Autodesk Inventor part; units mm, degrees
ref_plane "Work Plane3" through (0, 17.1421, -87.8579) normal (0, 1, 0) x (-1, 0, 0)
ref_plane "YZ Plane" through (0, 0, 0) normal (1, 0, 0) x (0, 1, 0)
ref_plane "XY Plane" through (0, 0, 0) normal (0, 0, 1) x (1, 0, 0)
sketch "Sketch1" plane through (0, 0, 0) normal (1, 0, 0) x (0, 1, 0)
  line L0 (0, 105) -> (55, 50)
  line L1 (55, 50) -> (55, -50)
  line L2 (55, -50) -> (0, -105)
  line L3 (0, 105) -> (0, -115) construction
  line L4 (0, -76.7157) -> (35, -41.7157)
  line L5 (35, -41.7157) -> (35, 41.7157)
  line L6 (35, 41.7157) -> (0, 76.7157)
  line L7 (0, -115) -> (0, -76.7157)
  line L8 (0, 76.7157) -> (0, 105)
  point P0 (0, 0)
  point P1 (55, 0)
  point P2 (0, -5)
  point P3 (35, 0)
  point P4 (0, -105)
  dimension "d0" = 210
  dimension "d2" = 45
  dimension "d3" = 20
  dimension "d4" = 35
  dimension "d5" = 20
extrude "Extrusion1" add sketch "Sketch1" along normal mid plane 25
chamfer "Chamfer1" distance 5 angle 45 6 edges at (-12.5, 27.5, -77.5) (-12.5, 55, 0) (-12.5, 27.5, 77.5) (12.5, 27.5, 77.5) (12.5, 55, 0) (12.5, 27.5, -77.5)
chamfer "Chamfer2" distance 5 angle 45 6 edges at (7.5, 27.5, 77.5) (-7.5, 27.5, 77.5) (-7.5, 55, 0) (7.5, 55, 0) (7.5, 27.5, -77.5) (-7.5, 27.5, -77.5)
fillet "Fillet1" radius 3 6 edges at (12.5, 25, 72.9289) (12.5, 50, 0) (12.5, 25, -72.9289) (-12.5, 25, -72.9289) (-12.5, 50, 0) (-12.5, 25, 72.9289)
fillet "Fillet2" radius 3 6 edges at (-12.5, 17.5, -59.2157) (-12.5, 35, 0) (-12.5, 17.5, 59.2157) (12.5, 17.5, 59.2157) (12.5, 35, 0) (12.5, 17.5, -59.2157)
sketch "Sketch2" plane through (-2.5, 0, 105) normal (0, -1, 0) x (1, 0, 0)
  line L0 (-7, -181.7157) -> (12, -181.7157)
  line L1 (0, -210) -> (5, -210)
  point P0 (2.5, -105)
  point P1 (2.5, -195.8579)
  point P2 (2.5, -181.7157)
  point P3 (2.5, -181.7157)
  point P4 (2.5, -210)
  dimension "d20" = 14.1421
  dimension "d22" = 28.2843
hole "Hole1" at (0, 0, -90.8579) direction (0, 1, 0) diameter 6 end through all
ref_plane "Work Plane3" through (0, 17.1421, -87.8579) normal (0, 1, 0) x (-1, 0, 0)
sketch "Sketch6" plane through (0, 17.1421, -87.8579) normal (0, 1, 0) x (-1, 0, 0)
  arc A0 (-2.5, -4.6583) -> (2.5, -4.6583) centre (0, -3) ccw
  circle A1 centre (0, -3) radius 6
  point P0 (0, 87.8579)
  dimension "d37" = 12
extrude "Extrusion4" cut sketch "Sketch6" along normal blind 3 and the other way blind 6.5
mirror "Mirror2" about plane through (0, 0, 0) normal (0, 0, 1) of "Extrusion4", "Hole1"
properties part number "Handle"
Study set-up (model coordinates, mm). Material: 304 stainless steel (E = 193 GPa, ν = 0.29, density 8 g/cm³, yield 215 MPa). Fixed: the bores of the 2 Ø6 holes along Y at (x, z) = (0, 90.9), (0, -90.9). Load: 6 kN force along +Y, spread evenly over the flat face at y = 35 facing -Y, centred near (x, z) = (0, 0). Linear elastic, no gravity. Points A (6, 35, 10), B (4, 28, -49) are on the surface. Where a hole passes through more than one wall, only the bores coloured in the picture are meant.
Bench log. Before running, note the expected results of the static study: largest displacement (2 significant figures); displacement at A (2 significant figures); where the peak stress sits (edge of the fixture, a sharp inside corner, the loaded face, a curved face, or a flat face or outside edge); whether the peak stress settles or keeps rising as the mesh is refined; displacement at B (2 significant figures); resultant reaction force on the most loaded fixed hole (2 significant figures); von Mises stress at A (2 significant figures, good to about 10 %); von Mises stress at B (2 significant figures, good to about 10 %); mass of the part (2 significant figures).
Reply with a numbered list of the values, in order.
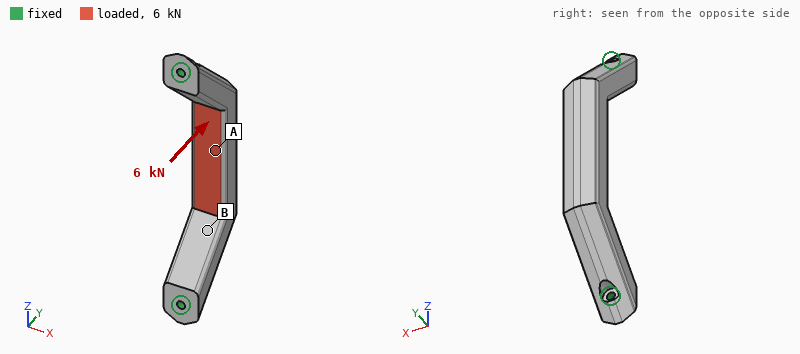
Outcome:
1. 23 µm
2. 22 µm
3. edge of the fixture
4. keeps rising
5. 7.1 µm
6. 5.0 kN
7. 17 MPa
8. 27 MPa
9. 770 g
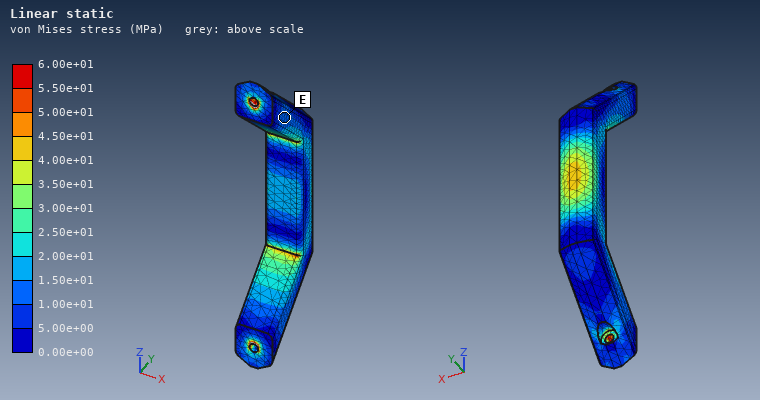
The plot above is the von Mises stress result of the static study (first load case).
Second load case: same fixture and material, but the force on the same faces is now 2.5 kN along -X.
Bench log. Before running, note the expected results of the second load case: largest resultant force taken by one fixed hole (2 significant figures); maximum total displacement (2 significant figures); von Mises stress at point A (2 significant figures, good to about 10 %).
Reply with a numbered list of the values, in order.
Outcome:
1. 1.3 kN
2. 63 µm
3. 13 MPa
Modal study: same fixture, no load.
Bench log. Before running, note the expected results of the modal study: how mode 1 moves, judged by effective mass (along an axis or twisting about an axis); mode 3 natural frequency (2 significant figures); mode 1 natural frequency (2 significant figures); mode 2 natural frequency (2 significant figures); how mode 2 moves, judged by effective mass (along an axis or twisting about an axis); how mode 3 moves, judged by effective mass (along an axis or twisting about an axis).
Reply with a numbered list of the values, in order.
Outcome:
1. along X
2. 4200 Hz
3. 1500 Hz
4. 3500 Hz
5. along Z
6. twisting about Y
